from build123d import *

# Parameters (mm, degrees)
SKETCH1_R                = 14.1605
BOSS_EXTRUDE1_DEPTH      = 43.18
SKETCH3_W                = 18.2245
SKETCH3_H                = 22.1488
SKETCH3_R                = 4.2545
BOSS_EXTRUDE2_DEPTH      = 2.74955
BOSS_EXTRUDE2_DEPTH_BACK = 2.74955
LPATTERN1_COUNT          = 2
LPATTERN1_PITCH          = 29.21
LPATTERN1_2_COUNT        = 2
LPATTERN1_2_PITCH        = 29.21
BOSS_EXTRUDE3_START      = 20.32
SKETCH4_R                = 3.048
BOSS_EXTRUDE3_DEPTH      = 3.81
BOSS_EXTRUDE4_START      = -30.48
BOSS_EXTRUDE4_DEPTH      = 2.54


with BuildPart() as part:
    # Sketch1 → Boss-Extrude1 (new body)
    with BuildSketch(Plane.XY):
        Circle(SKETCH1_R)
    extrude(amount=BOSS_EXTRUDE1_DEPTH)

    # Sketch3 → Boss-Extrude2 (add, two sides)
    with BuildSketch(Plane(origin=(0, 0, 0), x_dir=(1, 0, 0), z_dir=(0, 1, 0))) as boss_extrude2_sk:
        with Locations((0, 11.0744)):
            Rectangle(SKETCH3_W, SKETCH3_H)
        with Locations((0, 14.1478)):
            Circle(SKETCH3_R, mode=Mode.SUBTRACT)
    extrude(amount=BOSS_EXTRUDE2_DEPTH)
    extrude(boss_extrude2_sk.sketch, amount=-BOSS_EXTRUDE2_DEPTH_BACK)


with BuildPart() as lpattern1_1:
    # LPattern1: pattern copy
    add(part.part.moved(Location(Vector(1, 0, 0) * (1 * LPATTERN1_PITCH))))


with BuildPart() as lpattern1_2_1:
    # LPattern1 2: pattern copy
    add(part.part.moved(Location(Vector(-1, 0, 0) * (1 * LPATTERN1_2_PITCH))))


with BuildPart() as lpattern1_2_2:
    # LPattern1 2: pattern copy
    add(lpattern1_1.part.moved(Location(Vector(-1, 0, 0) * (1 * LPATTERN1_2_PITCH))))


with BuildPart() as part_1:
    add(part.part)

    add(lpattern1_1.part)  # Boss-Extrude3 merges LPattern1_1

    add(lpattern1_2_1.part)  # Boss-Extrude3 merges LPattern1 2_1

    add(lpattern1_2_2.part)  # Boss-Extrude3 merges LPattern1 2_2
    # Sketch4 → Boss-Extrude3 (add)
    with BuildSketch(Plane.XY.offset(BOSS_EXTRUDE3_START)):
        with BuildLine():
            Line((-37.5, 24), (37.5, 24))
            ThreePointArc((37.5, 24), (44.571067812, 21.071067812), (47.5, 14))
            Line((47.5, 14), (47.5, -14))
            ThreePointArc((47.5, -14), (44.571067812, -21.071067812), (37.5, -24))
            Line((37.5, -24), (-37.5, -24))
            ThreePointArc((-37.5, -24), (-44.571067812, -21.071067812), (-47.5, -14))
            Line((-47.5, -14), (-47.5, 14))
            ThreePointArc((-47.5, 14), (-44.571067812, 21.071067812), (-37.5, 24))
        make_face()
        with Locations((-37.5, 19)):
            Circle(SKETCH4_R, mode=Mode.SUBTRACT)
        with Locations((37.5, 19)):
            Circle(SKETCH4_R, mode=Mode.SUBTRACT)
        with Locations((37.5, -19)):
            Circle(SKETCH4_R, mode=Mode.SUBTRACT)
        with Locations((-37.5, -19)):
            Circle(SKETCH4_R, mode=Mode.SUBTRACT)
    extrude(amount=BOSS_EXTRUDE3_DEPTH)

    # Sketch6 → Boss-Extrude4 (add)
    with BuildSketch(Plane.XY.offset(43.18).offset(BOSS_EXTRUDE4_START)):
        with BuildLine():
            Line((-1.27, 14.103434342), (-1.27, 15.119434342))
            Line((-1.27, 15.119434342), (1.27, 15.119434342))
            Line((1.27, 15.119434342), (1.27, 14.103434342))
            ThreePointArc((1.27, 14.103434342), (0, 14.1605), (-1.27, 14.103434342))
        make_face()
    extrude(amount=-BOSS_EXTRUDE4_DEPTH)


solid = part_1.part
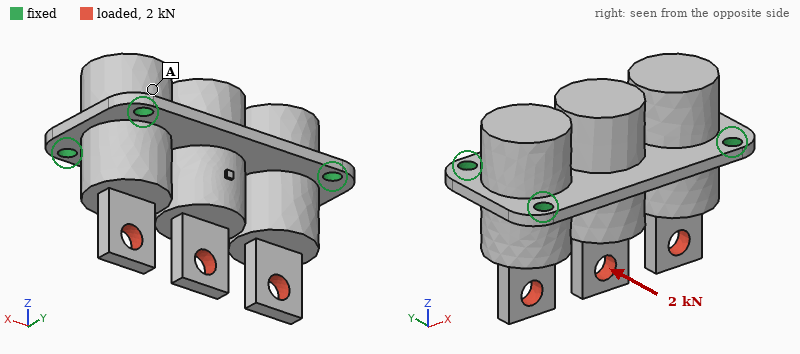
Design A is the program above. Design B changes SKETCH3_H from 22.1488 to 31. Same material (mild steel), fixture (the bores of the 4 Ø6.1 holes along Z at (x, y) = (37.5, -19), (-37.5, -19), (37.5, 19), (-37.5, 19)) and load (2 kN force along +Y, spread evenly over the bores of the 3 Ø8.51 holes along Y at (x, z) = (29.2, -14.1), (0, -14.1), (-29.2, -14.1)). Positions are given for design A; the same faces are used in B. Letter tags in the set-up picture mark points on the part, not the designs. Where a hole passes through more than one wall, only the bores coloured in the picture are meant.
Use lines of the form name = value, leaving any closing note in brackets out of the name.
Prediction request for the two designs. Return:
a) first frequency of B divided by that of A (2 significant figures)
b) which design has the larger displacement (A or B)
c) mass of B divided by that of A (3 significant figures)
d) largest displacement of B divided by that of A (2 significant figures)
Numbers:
first frequency of B divided by that of A = 0.97
which design has the larger displacement = B
mass of B divided by that of A = 1.01
largest displacement of B divided by that of A = 1.2
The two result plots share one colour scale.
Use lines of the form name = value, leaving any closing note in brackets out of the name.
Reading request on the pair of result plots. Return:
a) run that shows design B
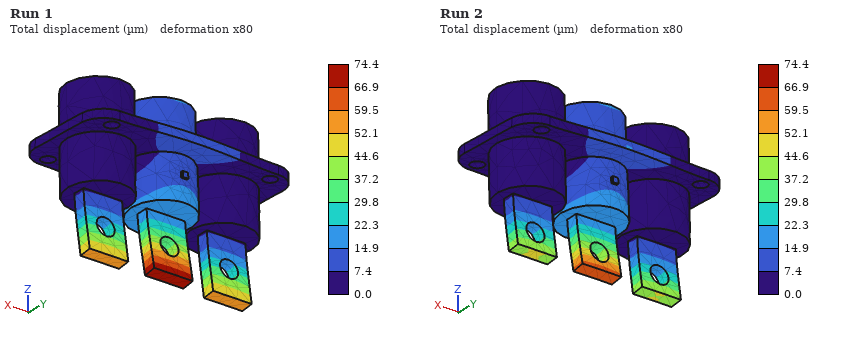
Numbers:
run that shows design B = Run 1
